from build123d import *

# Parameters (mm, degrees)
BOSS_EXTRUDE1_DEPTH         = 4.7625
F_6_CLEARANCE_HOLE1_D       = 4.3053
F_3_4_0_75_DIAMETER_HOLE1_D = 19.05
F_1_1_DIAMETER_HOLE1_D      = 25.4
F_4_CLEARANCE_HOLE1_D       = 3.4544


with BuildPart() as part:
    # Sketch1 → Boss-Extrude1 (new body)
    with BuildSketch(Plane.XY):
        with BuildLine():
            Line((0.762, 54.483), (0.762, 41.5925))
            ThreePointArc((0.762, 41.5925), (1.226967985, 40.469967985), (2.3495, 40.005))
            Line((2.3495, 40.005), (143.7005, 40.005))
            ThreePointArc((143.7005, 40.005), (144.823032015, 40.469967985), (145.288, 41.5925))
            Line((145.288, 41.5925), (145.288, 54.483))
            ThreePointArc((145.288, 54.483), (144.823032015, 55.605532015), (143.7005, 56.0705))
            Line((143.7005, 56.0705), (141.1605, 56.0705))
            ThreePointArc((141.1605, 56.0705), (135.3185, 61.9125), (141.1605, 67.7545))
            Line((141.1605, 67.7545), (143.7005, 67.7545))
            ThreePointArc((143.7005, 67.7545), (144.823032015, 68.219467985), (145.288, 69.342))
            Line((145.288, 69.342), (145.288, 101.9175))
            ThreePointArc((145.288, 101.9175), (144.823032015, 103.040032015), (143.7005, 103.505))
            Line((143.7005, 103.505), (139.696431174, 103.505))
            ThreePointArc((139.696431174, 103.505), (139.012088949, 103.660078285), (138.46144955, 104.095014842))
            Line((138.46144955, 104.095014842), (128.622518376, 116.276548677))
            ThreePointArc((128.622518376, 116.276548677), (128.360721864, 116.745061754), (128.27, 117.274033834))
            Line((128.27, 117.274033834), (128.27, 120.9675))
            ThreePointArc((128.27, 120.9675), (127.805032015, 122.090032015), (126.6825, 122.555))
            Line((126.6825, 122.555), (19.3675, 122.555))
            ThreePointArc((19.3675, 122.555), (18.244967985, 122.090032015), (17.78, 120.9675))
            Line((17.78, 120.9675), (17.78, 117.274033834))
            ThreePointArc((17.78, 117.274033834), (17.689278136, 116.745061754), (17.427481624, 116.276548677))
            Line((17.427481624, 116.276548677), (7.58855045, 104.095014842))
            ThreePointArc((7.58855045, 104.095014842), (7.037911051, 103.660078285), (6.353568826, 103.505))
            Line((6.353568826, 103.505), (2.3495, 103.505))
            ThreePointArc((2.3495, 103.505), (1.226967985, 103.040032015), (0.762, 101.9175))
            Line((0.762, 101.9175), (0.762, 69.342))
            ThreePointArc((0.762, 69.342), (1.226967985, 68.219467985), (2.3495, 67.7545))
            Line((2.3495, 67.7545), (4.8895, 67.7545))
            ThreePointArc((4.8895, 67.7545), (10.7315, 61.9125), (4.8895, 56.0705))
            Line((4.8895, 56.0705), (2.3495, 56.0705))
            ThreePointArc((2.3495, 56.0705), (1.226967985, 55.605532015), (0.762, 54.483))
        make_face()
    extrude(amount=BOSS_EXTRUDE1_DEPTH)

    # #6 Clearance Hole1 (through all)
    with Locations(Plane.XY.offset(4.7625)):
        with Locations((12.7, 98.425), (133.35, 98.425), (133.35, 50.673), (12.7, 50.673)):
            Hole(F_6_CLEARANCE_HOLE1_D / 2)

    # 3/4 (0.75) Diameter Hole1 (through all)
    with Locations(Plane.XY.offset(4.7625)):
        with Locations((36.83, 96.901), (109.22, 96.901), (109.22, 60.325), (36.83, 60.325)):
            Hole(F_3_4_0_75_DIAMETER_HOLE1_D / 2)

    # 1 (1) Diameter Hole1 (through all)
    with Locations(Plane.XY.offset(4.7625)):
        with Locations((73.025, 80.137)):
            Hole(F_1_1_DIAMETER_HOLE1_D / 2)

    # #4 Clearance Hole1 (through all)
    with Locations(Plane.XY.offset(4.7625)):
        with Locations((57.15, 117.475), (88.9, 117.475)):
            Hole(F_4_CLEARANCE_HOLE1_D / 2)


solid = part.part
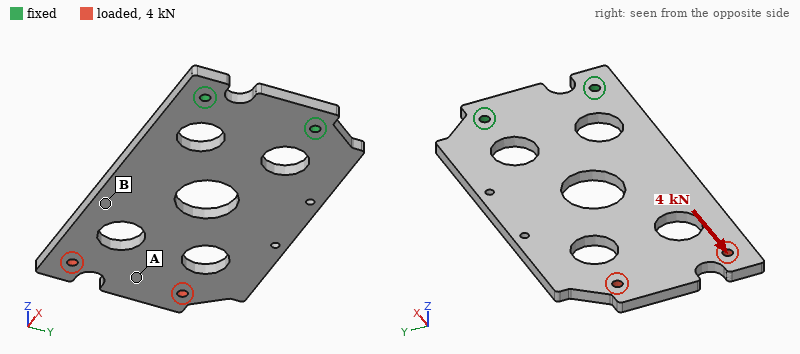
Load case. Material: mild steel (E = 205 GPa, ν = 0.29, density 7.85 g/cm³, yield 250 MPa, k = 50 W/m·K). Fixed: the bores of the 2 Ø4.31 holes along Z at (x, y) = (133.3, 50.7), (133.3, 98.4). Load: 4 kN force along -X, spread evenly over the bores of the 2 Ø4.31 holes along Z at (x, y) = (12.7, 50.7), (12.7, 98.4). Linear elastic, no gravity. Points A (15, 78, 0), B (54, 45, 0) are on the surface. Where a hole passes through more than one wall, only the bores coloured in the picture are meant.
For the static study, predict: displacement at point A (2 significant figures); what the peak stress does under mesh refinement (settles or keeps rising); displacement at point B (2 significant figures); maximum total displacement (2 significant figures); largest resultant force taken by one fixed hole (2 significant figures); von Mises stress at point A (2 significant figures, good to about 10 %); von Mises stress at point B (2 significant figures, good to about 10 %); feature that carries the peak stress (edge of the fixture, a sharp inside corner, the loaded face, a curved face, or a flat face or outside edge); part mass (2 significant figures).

11 µm
keeps rising
9.0 µm
15 µm
2.0 kN
6.7 MPa
22 MPa
edge of the fixture
350 g
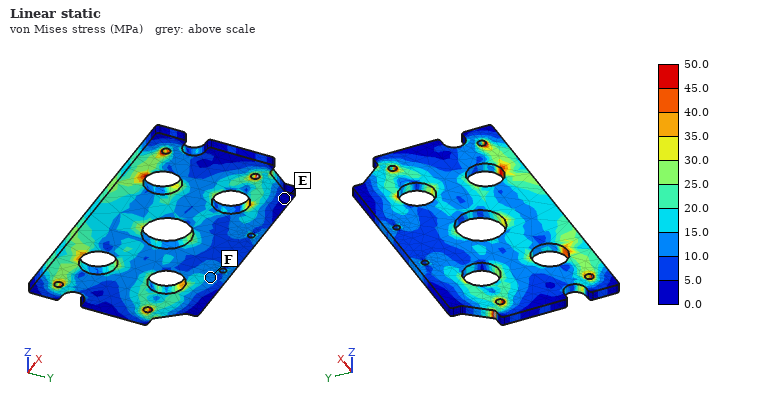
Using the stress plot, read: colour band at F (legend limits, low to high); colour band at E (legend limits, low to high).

10.0 to 15.0 MPa
0.0 to 5.0 MPa
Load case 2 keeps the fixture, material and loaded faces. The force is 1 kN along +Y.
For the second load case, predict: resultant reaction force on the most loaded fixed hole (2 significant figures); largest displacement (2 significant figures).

2.5 kN
45 µm
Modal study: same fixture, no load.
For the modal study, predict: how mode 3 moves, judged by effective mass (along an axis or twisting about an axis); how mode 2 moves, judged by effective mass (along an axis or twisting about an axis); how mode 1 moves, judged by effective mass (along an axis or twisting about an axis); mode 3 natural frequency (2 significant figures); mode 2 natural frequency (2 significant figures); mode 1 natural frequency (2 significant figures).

along Z
twisting about X
along Z
1300 Hz
740 Hz
200 Hz
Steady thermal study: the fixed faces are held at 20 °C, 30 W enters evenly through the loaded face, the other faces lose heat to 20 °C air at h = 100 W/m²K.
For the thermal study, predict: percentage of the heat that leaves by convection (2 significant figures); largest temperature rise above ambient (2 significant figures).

98 %
67 K
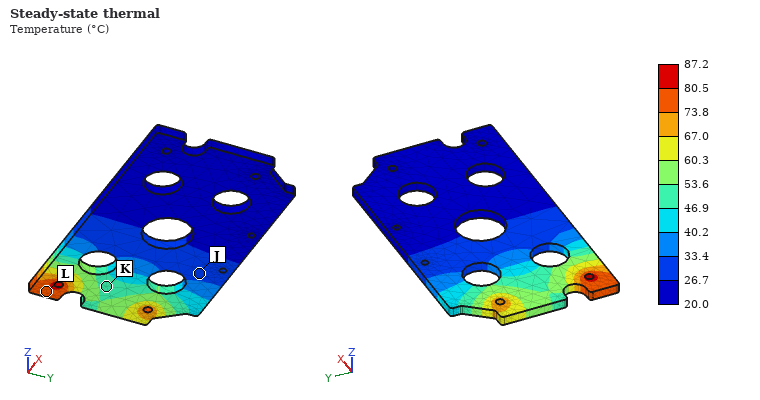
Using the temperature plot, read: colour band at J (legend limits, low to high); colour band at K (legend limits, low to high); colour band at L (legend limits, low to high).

26.7 to 33.4 °C
46.9 to 53.6 °C
73.8 to 80.5 °C
